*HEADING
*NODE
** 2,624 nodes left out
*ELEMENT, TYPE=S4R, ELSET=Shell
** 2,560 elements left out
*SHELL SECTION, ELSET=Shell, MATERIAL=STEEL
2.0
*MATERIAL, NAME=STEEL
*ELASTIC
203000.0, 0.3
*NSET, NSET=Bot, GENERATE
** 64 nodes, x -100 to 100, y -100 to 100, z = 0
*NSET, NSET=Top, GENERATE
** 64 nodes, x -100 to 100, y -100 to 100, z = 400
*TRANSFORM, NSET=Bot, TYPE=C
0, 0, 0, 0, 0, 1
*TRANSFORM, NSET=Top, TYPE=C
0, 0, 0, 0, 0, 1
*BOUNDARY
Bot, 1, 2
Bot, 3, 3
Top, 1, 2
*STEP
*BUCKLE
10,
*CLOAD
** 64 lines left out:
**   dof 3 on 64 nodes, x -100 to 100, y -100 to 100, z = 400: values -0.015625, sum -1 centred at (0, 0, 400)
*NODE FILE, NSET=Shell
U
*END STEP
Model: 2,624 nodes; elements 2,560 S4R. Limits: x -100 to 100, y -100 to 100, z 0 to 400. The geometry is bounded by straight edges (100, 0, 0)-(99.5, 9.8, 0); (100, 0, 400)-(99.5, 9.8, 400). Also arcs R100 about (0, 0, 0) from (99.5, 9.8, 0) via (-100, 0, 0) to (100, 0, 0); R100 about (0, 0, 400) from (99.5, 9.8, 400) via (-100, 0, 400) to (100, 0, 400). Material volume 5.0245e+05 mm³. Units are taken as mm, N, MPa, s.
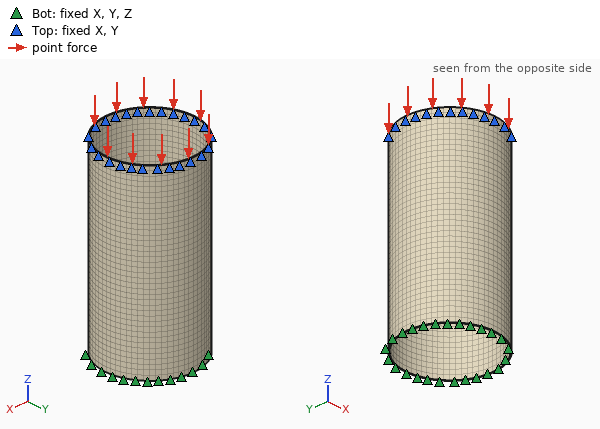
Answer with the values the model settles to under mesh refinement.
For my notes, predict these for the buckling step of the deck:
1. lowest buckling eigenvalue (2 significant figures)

2.9e+06
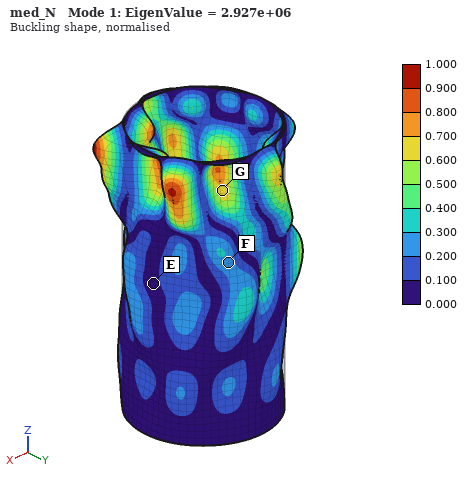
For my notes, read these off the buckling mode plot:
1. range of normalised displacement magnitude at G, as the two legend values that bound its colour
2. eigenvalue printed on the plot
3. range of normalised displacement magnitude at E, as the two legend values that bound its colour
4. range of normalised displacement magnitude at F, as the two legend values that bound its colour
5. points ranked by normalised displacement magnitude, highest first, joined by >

0.600 to 0.700
2.927e+06
0.000 to 0.100
0.200 to 0.300
G > F > E
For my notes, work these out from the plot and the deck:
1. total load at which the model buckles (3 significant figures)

2.93e+06 N
